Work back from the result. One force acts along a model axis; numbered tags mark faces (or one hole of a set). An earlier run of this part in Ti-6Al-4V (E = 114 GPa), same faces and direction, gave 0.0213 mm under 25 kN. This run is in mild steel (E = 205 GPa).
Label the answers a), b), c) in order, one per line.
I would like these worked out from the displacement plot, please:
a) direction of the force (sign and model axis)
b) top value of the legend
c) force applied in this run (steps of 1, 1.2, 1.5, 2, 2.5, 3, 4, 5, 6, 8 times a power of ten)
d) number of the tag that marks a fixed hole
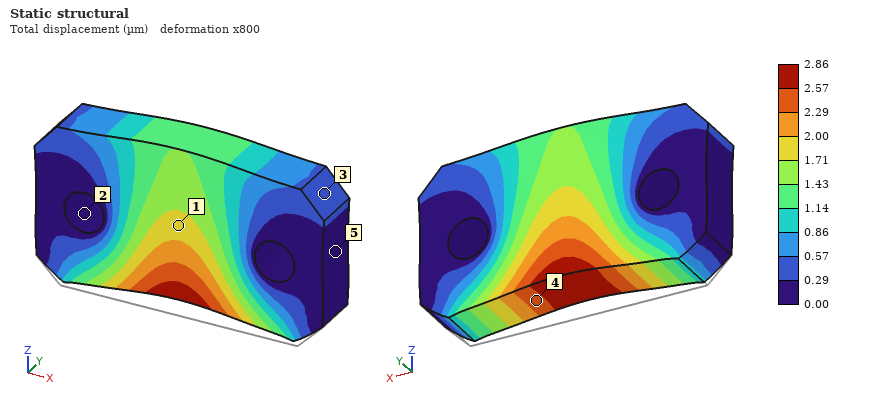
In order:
a) +Z
b) 2.86 µm
c) 6 kN
d) 2
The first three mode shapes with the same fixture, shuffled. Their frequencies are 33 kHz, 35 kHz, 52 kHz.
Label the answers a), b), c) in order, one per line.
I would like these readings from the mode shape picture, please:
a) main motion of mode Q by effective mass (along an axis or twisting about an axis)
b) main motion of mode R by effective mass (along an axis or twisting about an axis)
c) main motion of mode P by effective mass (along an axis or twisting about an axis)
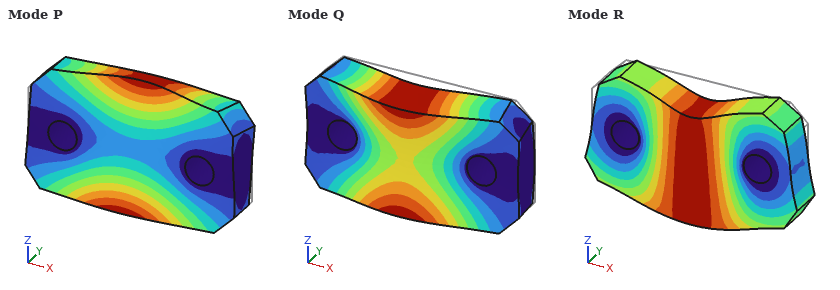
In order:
a) along Y
b) along Z
c) twisting about X
